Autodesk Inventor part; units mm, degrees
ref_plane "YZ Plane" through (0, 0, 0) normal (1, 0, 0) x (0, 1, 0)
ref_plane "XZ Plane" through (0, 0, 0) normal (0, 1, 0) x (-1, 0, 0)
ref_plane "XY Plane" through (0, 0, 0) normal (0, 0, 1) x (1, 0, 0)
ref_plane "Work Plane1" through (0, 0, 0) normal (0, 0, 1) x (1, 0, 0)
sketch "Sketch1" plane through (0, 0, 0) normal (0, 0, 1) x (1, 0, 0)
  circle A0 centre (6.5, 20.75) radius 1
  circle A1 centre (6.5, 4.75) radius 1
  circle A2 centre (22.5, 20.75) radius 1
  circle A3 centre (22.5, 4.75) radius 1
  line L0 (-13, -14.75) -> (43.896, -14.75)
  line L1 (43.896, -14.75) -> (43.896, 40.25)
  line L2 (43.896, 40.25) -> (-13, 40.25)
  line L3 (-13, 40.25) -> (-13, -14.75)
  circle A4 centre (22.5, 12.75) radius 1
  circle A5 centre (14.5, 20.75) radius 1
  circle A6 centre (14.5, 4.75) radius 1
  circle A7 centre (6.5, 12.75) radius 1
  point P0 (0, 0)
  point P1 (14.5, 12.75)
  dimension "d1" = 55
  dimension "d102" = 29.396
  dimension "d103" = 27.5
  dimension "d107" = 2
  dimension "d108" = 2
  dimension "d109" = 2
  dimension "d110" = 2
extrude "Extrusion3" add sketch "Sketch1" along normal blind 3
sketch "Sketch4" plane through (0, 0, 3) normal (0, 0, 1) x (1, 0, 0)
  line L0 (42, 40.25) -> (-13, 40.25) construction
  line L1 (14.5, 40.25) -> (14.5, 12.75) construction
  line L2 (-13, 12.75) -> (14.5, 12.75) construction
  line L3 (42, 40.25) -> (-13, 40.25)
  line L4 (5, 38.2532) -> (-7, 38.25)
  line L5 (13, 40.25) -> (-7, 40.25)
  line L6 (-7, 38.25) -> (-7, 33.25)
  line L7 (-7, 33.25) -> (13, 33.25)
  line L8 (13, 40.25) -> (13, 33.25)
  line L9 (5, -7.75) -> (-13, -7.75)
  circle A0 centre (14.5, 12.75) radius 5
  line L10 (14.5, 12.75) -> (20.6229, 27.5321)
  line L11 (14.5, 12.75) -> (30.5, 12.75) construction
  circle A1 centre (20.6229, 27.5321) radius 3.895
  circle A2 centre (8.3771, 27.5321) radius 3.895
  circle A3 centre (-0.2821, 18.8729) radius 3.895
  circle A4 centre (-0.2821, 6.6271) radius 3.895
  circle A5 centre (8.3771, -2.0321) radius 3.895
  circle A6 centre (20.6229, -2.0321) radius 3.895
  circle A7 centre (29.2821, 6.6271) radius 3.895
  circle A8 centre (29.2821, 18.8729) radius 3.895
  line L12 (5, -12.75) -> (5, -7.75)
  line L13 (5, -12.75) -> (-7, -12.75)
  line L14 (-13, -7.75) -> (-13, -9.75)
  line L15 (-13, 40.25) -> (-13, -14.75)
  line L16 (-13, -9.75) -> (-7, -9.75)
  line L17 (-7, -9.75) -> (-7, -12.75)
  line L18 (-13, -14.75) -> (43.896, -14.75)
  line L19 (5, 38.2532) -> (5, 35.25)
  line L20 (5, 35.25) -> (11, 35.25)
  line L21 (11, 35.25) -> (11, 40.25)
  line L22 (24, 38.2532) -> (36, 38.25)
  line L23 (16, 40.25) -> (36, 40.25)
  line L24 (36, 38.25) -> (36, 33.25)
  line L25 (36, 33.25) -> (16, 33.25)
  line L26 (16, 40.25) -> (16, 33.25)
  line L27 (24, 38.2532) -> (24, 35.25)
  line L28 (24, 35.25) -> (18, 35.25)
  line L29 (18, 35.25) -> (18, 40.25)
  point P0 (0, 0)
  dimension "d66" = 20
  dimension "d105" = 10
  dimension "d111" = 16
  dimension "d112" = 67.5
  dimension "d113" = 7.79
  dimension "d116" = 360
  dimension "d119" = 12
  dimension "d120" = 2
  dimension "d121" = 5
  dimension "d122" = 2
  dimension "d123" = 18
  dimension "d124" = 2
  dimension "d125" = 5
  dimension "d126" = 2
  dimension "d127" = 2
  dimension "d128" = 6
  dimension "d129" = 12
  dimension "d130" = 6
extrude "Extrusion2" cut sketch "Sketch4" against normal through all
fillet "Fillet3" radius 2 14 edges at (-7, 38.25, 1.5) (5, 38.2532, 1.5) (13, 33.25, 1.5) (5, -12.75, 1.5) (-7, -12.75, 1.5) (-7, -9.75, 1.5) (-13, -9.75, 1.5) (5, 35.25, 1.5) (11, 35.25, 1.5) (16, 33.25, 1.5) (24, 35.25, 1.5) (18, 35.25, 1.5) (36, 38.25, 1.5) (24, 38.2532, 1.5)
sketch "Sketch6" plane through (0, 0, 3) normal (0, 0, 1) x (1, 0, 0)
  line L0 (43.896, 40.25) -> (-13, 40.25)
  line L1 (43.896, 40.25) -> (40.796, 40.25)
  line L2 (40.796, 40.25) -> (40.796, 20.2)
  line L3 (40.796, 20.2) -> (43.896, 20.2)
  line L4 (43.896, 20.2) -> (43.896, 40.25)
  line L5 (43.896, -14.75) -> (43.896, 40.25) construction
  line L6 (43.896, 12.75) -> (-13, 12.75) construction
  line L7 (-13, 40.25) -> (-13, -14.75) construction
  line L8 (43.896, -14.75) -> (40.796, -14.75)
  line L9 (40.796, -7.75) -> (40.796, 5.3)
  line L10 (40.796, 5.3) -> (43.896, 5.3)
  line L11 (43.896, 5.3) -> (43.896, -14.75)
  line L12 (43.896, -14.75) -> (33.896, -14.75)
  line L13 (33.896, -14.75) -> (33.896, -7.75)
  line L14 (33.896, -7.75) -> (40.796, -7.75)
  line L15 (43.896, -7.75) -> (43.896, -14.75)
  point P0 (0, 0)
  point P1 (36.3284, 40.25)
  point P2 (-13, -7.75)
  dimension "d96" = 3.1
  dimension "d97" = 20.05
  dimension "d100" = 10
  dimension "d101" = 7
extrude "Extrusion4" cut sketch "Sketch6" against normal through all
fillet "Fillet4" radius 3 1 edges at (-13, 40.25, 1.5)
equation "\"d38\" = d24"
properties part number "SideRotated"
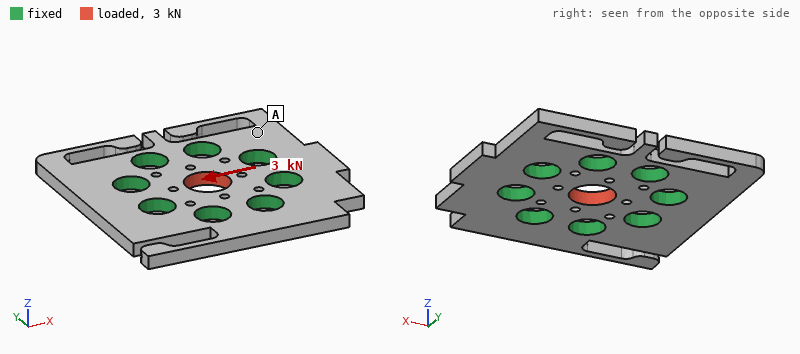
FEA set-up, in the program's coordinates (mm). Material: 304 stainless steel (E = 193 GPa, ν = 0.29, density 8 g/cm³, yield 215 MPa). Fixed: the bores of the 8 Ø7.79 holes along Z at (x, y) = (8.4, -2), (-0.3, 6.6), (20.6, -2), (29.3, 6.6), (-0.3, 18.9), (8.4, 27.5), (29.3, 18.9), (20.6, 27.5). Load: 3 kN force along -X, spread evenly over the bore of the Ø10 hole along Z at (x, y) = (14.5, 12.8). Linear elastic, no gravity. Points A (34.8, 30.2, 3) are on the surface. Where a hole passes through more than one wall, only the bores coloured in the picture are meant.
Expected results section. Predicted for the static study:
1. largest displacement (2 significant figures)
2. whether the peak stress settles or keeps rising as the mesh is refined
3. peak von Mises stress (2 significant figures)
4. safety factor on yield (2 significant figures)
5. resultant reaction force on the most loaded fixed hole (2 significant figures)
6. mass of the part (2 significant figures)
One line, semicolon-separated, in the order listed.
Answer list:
1.4 µm; settles; 85 MPa; 2.5; 620 N; 53 g
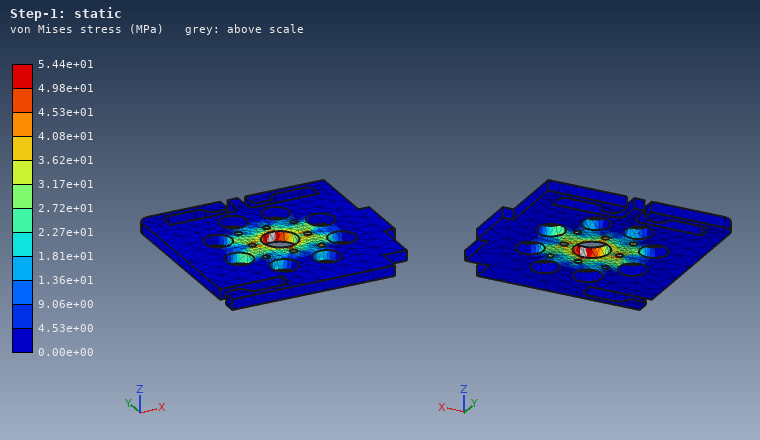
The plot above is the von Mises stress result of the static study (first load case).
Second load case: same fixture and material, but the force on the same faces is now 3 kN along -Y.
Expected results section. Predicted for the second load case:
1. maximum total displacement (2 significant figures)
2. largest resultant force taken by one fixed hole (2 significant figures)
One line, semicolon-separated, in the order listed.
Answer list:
1.4 µm; 620 N
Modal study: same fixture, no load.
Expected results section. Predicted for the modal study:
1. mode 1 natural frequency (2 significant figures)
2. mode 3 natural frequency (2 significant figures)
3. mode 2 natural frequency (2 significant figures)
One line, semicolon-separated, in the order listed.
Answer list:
3100 Hz; 3200 Hz; 3200 Hz
